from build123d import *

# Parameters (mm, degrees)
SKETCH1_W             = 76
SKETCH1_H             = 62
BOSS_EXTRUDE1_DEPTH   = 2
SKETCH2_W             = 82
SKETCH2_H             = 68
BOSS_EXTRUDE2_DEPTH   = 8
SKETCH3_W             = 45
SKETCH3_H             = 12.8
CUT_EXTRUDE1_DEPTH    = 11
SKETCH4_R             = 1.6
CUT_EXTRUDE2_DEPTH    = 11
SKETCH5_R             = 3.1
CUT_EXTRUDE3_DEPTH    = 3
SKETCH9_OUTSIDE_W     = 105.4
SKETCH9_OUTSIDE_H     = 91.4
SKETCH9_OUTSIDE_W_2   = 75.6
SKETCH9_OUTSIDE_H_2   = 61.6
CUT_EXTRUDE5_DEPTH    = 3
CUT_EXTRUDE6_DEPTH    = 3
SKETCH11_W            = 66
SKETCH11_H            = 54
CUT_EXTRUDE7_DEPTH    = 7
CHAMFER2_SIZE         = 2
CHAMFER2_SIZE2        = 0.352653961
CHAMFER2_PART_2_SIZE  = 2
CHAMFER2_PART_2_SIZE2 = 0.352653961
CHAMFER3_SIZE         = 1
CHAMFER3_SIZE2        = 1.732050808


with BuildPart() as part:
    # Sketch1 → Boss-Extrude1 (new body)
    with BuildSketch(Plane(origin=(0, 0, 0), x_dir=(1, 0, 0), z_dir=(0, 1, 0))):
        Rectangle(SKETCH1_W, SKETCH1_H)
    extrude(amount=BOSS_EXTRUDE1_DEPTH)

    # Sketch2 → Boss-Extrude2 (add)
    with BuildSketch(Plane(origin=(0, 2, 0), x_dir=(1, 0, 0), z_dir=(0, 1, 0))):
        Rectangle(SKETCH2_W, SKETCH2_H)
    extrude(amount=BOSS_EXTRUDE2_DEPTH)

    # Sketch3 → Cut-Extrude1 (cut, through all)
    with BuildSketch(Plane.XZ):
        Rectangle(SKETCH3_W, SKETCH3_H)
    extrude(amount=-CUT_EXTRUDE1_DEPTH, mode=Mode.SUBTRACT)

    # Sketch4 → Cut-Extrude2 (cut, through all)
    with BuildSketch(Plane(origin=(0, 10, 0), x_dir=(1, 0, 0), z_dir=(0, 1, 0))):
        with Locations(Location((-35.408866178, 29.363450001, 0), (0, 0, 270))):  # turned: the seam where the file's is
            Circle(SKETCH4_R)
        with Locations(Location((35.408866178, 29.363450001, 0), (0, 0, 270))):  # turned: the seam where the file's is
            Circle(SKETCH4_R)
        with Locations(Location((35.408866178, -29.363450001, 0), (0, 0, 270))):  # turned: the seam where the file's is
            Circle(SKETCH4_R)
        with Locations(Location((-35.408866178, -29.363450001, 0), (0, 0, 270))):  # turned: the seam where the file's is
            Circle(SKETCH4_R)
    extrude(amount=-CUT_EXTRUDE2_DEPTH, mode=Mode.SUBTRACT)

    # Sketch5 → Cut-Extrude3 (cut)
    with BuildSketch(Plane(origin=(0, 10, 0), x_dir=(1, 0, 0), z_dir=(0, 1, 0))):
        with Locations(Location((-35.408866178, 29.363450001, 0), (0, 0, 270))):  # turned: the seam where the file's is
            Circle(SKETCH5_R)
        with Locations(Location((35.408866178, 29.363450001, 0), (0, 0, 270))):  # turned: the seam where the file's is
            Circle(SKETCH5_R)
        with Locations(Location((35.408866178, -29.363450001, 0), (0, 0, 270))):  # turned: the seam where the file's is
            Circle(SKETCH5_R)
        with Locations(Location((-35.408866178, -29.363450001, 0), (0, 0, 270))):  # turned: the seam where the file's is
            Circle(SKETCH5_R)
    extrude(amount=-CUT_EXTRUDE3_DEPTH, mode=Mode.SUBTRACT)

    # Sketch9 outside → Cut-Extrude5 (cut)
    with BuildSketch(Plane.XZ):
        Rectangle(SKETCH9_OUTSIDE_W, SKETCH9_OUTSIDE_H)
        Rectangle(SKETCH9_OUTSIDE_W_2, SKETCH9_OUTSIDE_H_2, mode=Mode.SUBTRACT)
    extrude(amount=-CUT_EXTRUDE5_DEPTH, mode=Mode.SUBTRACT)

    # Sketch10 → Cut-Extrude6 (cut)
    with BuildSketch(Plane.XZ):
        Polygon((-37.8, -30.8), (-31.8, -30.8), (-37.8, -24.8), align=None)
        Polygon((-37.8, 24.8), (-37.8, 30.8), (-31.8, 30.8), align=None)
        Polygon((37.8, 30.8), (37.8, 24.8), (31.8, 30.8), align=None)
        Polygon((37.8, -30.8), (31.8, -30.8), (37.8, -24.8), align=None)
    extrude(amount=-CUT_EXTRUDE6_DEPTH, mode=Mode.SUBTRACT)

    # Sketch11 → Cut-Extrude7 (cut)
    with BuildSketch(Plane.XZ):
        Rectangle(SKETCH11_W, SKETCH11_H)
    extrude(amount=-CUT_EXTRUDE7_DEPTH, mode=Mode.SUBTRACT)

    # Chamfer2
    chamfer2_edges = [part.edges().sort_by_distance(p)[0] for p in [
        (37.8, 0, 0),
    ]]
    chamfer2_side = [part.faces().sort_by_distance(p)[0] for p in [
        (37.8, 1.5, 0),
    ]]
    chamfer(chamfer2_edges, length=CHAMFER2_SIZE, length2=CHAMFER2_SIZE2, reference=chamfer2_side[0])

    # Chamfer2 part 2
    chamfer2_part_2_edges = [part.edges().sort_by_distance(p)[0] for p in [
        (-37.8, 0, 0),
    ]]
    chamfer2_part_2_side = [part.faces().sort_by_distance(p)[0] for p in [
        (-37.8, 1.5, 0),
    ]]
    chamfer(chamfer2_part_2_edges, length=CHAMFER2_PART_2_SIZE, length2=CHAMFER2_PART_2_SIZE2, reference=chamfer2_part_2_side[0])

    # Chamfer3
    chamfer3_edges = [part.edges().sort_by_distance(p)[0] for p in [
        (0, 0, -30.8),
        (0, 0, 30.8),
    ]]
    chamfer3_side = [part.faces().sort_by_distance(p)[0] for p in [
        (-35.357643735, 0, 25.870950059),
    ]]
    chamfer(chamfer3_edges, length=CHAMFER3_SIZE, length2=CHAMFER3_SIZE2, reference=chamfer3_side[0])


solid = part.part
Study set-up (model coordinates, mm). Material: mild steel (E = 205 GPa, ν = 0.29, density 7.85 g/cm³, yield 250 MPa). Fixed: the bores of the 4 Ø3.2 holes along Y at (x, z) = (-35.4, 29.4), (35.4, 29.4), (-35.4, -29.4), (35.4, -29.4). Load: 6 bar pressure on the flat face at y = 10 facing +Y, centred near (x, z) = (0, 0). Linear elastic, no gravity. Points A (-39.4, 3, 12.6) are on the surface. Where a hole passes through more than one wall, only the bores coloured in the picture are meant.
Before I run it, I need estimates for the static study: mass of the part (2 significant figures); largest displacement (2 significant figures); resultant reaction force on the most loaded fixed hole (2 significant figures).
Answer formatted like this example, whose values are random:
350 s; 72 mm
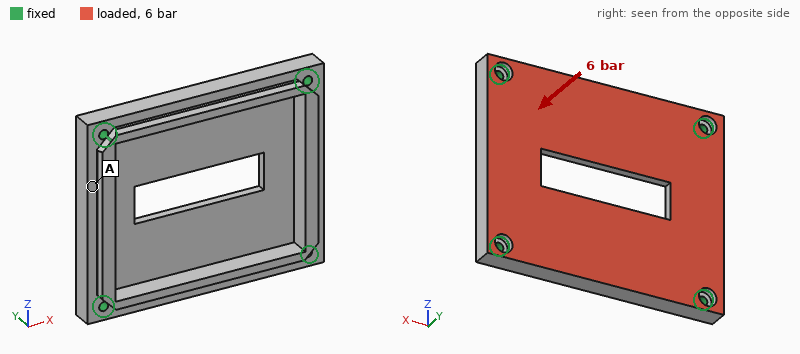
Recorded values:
200 g; 55 µm; 960 N
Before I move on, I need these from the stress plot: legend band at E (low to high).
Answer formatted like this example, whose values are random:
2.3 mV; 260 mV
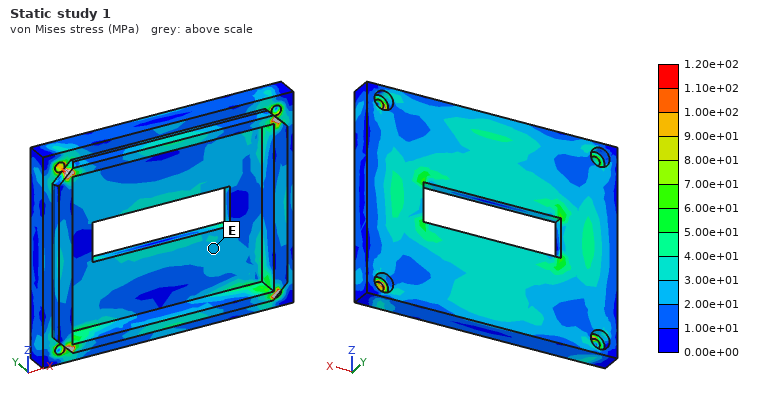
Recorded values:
2.00e+01 to 3.00e+01 MPa
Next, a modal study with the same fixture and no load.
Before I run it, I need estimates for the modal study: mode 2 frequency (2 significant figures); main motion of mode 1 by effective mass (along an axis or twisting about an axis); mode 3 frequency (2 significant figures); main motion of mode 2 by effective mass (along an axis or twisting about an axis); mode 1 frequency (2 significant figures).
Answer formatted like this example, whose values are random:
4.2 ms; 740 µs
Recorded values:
5500 Hz; along Y; 8100 Hz; twisting about X; 4600 Hz
